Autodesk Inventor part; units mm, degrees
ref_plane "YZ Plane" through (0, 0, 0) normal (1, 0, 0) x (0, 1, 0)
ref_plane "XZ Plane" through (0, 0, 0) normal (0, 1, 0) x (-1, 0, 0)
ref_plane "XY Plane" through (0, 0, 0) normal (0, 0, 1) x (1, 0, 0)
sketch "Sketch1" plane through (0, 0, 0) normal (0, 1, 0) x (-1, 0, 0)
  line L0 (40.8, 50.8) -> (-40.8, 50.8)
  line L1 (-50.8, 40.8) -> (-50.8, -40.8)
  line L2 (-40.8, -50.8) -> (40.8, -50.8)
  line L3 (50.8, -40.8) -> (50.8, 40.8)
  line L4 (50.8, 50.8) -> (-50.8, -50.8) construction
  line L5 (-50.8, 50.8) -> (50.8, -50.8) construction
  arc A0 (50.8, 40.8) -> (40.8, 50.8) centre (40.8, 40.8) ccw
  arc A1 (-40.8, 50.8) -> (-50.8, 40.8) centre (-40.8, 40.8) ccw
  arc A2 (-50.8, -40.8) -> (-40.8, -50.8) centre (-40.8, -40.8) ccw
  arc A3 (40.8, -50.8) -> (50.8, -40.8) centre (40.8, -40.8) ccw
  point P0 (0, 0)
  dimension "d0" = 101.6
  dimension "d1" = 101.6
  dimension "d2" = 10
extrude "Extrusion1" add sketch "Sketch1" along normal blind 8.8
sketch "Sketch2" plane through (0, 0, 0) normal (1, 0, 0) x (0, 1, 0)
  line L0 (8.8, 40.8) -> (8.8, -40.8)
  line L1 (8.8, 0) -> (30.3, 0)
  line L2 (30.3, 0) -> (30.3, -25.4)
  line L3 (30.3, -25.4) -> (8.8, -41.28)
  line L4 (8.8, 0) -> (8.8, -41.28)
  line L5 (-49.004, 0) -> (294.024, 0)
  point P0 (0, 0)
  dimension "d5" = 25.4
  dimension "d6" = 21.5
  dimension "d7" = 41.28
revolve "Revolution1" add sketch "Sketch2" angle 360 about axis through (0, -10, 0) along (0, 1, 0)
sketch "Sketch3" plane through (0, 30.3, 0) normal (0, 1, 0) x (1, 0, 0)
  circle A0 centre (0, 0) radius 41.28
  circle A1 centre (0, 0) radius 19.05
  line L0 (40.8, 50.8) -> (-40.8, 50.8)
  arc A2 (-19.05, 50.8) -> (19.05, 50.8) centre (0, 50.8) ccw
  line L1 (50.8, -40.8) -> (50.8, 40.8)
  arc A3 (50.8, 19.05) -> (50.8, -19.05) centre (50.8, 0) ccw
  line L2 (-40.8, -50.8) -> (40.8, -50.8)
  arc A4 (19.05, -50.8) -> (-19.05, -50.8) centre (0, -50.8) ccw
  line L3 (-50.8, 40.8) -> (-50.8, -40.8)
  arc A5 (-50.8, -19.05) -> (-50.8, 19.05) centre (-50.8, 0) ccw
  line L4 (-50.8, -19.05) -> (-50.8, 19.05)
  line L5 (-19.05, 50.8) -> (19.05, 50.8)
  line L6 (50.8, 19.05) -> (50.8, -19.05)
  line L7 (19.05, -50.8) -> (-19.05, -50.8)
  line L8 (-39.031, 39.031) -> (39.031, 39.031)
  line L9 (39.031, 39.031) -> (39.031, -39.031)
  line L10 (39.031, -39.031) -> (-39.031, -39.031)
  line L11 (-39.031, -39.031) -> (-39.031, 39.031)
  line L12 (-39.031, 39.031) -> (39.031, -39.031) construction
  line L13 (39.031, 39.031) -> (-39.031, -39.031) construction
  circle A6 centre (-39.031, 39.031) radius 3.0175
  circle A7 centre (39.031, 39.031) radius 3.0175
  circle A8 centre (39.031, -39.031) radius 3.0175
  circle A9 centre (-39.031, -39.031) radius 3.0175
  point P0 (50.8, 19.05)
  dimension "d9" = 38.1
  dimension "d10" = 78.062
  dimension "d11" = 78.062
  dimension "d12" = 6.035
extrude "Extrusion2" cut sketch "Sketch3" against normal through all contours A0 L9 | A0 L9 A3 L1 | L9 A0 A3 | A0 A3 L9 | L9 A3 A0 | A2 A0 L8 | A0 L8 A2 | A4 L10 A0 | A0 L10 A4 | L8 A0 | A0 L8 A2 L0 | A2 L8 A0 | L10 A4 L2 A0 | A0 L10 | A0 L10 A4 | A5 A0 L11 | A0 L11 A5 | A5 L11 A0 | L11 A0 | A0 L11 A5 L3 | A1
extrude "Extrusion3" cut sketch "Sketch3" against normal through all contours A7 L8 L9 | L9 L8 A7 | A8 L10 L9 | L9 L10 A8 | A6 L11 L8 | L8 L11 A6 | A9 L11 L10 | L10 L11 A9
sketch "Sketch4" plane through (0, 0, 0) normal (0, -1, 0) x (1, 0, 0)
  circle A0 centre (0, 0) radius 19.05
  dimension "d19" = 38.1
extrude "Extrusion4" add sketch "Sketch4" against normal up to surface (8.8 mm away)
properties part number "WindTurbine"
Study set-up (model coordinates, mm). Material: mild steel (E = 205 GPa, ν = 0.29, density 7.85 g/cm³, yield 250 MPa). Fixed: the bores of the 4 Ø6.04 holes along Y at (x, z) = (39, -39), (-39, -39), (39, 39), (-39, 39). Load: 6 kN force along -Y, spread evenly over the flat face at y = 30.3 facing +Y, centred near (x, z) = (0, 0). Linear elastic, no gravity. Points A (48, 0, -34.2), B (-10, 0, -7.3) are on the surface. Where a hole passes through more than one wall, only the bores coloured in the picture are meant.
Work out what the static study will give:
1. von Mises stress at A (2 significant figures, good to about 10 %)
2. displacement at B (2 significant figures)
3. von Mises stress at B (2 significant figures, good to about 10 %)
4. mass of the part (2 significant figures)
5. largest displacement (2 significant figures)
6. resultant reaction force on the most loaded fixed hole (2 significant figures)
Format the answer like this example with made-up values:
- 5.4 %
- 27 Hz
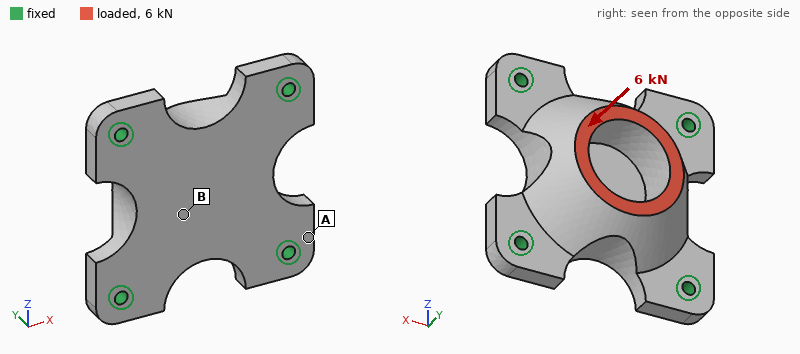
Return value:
- 13 MPa
- 6.8 µm
- 5.1 MPa
- 920 g
- 7.0 µm
- 1.8 kN
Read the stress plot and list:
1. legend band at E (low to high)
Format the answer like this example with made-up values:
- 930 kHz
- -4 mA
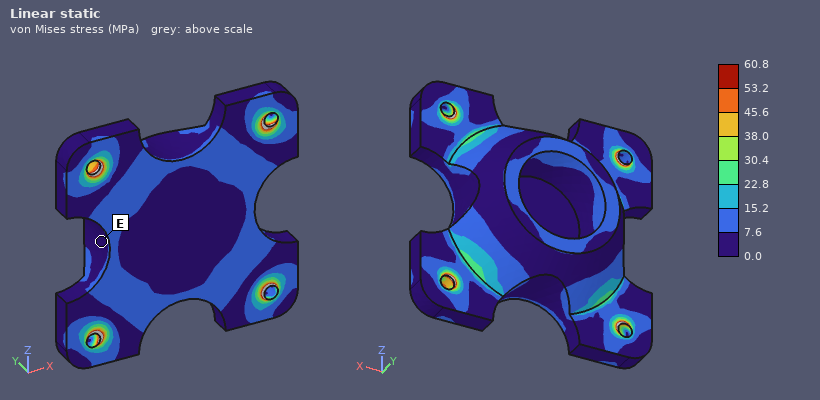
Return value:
- 0.0 to 7.6 MPa
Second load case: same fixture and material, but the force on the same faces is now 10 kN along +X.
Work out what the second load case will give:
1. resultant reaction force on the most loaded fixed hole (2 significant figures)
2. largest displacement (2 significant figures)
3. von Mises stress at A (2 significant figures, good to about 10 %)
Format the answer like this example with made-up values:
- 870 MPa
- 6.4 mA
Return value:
- 3.5 kN
- 11 µm
- 21 MPa
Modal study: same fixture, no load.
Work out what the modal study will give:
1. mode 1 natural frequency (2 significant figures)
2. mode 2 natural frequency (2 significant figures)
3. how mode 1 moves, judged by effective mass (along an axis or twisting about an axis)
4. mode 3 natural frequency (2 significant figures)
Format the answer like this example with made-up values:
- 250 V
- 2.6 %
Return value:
- 5900 Hz
- 9000 Hz
- along Y
- 9000 Hz
